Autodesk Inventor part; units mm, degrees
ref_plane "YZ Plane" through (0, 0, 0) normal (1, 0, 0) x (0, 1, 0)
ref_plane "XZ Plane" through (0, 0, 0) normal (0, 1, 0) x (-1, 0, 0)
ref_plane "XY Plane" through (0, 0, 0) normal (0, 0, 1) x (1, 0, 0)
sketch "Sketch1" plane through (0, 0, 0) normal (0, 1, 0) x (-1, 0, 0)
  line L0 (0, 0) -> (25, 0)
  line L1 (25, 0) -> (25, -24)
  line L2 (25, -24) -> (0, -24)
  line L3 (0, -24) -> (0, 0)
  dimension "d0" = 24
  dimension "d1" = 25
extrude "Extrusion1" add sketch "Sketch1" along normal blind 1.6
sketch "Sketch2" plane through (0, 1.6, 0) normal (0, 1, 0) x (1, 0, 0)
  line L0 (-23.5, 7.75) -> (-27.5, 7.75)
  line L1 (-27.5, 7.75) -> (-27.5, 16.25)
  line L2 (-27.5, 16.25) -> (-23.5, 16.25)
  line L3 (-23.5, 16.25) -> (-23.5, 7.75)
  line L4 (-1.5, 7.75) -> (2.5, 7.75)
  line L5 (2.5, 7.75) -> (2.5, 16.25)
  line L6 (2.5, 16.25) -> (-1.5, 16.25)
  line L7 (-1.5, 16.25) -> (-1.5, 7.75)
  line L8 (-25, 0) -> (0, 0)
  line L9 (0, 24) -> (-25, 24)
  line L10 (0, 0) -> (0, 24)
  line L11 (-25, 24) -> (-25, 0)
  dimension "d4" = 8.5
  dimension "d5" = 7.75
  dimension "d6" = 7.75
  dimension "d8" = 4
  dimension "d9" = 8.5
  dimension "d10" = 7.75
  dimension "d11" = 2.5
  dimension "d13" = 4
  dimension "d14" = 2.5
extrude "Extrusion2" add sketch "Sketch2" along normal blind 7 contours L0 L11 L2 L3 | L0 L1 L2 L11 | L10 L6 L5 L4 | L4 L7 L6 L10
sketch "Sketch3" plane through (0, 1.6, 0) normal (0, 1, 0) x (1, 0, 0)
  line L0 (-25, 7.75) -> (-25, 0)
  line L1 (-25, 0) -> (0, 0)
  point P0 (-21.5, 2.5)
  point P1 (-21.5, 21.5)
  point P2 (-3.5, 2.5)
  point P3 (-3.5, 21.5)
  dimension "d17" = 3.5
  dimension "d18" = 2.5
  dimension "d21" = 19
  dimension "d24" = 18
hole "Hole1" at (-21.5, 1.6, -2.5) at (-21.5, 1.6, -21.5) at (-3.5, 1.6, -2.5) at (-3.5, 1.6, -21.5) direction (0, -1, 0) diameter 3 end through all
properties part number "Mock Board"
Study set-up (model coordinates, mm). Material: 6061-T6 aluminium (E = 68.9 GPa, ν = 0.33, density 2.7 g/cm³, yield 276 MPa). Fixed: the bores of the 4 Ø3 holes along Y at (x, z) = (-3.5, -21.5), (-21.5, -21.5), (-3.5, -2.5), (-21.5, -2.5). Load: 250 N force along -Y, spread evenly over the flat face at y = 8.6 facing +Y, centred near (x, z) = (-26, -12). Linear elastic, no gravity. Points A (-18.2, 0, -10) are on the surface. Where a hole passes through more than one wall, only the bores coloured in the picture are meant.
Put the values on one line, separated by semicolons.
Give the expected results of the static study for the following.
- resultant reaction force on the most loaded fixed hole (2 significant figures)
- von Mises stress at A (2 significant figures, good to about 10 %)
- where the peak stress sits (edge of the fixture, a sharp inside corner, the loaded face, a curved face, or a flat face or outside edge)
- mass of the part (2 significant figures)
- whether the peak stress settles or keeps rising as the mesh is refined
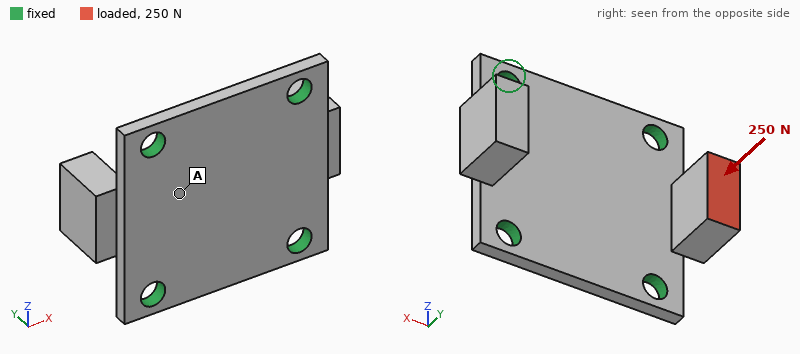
150 N; 35 MPa; edge of the fixture; 3.8 g; keeps rising
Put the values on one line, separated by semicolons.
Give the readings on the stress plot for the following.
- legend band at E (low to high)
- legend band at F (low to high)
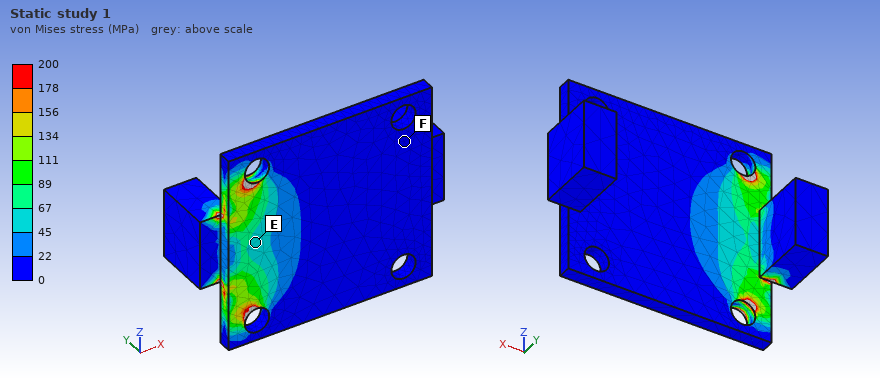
45 to 67 MPa; 0 to 22 MPa
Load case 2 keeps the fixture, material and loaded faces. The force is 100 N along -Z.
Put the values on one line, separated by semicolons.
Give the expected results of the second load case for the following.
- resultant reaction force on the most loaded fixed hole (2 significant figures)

81 N
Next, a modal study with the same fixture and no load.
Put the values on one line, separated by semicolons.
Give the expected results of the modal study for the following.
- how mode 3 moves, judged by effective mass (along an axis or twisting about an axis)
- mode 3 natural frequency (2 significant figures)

along Y; 19 kHz
